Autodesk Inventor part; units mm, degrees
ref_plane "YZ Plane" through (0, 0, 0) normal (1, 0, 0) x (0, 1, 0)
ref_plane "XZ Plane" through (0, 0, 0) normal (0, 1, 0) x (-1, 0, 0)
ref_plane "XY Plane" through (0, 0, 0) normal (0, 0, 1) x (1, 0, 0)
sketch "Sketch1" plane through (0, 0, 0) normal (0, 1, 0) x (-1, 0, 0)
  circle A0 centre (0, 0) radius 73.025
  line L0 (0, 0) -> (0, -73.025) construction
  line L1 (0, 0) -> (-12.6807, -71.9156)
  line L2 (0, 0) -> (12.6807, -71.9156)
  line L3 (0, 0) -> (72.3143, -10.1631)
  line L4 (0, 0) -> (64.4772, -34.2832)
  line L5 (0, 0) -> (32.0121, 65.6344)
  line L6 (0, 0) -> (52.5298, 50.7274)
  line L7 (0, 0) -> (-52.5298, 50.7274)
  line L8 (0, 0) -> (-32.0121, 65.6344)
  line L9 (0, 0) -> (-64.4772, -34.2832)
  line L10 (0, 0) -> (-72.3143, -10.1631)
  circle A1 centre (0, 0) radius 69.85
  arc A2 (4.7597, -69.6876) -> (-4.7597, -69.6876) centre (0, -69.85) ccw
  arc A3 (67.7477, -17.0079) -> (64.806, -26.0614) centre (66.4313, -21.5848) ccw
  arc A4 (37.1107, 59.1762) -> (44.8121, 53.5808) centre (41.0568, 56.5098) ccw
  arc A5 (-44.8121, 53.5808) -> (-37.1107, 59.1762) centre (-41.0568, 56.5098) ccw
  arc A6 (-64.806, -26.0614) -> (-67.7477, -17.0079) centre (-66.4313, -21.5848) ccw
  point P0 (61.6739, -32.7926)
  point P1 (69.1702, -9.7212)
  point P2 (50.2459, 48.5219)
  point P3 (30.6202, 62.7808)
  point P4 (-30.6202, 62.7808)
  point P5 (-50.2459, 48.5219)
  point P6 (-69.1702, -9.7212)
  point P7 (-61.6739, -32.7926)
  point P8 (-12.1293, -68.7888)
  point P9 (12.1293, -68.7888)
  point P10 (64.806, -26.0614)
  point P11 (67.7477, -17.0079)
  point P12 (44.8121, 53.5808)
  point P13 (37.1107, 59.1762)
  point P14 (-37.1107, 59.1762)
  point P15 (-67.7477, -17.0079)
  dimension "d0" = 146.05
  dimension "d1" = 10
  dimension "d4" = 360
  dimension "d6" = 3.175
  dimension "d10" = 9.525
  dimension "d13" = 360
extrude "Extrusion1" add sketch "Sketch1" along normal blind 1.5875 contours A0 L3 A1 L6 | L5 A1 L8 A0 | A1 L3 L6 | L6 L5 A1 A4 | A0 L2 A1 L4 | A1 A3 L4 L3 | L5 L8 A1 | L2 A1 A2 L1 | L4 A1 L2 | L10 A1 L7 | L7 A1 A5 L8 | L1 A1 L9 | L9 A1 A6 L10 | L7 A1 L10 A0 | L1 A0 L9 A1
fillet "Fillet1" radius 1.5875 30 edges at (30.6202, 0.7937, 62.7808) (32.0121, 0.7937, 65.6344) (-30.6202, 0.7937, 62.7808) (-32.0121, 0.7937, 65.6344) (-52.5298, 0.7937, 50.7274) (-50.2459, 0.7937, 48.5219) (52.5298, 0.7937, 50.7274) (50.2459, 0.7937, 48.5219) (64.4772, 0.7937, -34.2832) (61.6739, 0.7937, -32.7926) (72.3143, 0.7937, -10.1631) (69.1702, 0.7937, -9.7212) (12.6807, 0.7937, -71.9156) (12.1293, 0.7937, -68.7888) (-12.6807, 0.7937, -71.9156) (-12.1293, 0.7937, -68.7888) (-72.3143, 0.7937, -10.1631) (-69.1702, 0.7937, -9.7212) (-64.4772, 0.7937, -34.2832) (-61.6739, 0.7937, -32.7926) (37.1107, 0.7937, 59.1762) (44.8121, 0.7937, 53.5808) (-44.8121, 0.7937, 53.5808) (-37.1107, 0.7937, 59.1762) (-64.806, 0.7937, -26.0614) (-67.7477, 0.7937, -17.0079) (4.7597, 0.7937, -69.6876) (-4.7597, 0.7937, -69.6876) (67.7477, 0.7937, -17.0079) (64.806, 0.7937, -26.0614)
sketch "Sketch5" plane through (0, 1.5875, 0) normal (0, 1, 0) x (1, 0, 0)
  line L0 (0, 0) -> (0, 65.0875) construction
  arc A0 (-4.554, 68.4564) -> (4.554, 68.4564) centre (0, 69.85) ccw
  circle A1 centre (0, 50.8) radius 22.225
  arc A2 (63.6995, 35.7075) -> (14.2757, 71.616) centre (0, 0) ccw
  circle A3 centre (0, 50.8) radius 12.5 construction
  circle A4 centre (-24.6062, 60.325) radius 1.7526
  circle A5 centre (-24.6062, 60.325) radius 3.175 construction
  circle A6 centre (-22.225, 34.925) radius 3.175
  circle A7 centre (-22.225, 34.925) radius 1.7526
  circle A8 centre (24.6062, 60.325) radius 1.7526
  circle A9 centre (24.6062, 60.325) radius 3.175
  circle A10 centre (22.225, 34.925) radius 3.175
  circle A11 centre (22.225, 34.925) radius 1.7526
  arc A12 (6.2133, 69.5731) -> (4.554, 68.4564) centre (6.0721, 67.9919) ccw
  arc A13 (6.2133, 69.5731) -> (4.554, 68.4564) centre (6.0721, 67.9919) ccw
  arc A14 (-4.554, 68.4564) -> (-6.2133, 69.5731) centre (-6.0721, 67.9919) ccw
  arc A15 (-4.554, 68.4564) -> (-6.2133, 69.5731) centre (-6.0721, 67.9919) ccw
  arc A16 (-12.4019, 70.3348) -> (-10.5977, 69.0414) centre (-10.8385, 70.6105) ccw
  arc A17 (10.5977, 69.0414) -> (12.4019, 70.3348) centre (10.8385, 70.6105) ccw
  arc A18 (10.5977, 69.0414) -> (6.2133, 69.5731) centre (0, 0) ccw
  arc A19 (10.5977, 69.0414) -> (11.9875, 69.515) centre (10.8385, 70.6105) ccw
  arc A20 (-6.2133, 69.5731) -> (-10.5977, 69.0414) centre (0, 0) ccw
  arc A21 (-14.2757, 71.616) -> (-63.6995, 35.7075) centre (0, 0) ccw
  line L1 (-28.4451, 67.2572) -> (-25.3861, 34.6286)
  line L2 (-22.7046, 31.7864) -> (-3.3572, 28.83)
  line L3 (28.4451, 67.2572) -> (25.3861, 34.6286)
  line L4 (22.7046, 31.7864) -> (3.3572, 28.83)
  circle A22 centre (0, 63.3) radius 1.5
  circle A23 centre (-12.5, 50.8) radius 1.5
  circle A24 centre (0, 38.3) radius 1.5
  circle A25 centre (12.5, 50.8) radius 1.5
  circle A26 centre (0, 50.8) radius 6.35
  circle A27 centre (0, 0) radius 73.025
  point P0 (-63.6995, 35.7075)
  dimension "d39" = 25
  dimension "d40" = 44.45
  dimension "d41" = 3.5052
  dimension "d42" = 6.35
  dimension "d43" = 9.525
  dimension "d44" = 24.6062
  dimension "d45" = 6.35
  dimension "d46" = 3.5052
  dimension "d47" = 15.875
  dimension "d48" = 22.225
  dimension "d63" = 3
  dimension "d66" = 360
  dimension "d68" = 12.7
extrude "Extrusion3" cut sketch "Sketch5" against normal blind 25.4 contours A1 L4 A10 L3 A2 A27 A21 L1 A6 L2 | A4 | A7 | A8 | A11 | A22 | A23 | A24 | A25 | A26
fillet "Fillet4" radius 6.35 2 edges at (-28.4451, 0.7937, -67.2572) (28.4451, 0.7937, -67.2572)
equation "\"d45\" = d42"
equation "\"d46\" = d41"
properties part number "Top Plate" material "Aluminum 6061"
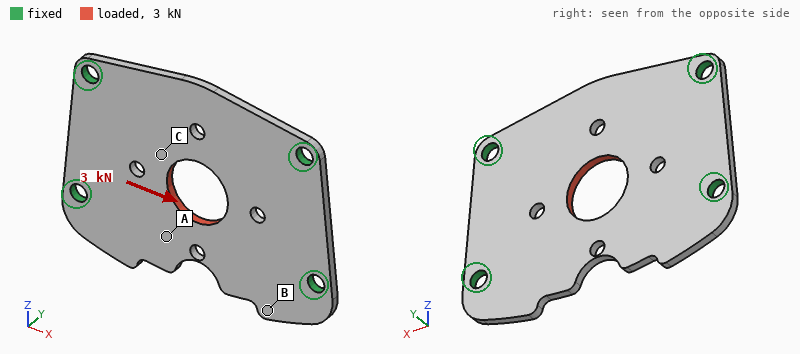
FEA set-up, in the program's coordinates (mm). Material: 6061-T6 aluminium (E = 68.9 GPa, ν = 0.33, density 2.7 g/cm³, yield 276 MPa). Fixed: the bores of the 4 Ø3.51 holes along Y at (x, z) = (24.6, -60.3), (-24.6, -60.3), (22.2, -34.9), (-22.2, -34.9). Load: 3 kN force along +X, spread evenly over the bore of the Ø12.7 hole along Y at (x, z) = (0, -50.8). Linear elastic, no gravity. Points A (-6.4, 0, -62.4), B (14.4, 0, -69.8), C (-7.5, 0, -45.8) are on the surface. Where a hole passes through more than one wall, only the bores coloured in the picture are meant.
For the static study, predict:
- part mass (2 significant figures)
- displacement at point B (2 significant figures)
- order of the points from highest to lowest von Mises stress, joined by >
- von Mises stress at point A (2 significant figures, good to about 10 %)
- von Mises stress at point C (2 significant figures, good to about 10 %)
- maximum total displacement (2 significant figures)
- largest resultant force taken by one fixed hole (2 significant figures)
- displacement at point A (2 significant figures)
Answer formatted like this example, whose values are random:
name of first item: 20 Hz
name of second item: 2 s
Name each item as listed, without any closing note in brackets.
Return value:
part mass: 8.0 g
displacement at point B: 6.6 µm
order of the points from highest to lowest von Mises stress, joined by >: C > A > B
von Mises stress at point A: 20 MPa
von Mises stress at point C: 44 MPa
maximum total displacement: 15 µm
largest resultant force taken by one fixed hole: 880 N
displacement at point A: 8.8 µm
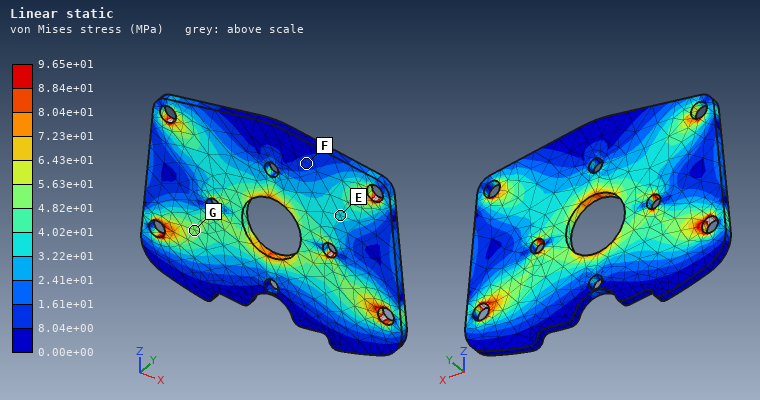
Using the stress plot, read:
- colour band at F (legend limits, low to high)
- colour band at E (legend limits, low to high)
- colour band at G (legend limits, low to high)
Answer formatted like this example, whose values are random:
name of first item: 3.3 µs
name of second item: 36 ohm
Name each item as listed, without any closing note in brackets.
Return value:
colour band at F: 8.04e+00 to 1.61e+01 MPa
colour band at E: 3.22e+01 to 4.02e+01 MPa
colour band at G: 4.82e+01 to 5.63e+01 MPa
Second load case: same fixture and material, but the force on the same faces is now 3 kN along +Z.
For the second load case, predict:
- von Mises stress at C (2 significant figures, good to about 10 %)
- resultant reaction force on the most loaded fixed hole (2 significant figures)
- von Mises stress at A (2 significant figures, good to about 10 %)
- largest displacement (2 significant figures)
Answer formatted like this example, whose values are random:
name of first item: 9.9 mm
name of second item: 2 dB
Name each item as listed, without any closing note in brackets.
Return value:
von Mises stress at C: 54 MPa
resultant reaction force on the most loaded fixed hole: 1.1 kN
von Mises stress at A: 35 MPa
largest displacement: 41 µm
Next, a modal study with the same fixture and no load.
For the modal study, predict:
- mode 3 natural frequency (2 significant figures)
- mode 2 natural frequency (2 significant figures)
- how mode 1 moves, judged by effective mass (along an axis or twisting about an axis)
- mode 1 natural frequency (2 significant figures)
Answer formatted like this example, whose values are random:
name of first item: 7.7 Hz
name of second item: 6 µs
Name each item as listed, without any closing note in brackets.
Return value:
mode 3 natural frequency: 7600 Hz
mode 2 natural frequency: 4800 Hz
how mode 1 moves, judged by effective mass: along Y
mode 1 natural frequency: 3600 Hz
